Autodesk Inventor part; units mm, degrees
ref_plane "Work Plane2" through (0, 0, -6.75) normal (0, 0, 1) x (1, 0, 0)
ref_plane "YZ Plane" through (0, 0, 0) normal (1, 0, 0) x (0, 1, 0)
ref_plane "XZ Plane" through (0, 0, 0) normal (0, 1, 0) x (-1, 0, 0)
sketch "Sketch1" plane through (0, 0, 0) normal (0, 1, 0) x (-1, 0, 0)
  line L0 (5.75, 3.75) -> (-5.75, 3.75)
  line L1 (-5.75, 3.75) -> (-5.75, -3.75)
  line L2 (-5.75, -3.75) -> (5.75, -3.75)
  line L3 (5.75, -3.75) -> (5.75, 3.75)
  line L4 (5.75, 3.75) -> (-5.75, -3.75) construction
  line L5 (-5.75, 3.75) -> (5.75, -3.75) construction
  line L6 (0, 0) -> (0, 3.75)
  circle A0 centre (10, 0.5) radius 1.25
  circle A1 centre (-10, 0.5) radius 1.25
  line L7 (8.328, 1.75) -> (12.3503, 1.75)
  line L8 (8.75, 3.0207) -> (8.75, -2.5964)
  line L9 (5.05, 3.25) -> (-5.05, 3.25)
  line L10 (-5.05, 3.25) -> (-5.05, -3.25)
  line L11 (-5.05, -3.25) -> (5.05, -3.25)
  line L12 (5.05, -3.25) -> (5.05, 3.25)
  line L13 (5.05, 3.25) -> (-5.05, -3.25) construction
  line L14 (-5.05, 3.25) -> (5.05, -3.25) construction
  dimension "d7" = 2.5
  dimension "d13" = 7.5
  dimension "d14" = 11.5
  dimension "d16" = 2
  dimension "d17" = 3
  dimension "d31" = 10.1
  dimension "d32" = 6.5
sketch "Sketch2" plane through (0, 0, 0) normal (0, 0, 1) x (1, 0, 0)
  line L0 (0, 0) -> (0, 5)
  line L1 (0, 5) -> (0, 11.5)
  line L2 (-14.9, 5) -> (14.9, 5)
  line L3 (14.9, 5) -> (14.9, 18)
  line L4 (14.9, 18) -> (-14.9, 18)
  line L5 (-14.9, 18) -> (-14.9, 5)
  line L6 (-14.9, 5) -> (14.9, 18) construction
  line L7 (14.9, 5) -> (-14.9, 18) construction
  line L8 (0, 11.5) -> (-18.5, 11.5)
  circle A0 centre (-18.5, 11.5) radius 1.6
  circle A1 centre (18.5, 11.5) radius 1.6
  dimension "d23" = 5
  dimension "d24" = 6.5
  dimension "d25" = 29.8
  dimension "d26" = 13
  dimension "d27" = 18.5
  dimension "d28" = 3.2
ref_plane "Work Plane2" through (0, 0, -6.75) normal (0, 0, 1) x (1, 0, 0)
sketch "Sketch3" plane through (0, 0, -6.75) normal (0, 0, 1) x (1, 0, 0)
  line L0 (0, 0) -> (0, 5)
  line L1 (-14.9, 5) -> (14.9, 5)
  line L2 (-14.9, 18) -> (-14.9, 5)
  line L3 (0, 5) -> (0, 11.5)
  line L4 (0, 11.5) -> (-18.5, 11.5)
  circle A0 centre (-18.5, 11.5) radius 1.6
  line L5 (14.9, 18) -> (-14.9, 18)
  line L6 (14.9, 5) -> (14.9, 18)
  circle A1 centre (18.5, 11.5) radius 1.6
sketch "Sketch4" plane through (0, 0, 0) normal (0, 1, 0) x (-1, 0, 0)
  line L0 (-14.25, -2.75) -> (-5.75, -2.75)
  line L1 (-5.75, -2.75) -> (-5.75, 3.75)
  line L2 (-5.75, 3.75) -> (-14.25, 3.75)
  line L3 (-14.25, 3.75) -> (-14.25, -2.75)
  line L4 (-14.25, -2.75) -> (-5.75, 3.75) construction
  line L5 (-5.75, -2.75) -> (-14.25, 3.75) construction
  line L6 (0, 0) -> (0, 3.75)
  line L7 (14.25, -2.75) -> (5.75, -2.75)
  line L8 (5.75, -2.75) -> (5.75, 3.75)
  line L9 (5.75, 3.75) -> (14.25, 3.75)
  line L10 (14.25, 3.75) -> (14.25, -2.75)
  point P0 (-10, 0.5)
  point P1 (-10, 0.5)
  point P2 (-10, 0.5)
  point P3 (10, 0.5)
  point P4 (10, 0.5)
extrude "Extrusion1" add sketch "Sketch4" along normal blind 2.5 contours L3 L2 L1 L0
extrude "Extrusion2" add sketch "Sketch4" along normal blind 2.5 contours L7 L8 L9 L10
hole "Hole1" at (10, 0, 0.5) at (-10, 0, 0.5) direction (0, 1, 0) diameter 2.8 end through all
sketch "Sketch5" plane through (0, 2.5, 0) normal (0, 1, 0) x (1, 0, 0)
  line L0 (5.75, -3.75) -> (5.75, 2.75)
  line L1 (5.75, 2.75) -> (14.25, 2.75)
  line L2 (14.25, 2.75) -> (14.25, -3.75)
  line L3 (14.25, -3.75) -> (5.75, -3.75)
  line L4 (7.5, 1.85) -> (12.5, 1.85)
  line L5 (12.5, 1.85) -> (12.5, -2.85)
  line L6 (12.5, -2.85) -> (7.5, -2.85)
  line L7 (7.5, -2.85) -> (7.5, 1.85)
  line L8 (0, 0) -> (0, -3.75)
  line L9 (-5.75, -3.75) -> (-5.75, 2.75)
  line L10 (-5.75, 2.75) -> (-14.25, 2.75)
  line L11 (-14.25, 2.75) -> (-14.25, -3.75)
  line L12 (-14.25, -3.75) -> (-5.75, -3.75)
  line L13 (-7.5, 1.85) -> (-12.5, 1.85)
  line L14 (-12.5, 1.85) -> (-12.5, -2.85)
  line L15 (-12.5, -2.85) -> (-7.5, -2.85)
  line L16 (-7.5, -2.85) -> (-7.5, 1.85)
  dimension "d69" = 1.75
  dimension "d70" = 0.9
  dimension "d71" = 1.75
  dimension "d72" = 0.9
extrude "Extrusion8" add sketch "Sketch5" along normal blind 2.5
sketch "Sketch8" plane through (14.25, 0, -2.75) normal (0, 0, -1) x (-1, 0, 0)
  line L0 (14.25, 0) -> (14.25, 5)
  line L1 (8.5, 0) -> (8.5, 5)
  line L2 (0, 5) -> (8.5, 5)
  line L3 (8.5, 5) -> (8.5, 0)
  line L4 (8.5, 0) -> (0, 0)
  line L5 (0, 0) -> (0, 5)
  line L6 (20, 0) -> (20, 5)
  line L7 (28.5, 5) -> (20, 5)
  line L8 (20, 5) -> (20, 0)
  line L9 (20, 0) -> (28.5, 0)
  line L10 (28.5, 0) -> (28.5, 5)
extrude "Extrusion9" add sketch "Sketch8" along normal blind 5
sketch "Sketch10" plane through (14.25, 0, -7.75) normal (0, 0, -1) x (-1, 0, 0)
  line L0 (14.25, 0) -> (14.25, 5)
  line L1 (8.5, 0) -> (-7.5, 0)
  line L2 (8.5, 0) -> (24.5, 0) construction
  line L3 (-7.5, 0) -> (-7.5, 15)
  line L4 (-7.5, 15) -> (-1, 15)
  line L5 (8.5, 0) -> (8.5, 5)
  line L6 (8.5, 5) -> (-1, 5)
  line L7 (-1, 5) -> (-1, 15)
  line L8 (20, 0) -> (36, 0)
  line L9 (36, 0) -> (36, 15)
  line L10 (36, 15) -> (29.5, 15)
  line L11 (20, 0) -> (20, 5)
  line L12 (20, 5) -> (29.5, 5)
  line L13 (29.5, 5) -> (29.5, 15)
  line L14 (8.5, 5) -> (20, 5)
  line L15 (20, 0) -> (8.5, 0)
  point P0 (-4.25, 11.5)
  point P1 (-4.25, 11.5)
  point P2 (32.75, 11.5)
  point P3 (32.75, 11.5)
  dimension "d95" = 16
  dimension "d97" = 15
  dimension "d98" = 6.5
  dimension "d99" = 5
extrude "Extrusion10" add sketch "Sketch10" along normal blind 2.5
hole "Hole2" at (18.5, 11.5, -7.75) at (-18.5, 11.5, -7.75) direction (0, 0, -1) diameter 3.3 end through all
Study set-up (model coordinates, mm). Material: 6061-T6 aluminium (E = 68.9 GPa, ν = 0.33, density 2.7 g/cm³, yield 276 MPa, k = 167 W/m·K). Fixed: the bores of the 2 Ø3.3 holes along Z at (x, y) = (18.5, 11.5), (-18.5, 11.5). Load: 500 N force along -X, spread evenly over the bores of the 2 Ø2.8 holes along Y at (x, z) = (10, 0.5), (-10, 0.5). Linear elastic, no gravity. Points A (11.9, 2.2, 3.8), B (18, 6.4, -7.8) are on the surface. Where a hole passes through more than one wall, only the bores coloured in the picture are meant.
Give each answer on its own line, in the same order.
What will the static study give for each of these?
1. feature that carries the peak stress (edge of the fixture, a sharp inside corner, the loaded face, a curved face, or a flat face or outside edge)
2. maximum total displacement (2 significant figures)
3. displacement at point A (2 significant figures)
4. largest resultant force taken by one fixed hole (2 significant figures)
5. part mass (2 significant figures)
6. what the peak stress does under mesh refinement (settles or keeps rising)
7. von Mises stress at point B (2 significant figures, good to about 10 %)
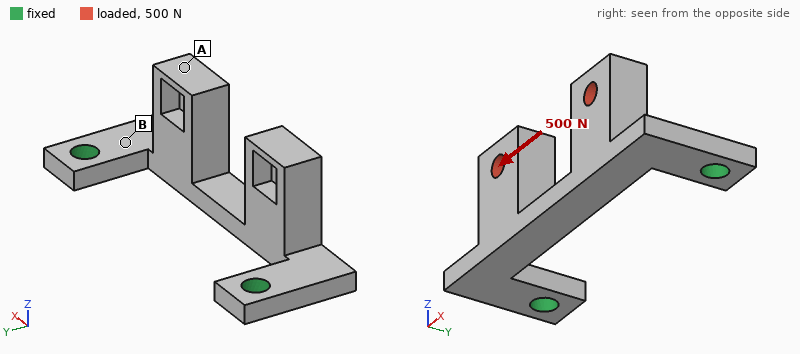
edge of the fixture
96 µm
90 µm
290 N
4.5 g
keeps rising
62 MPa
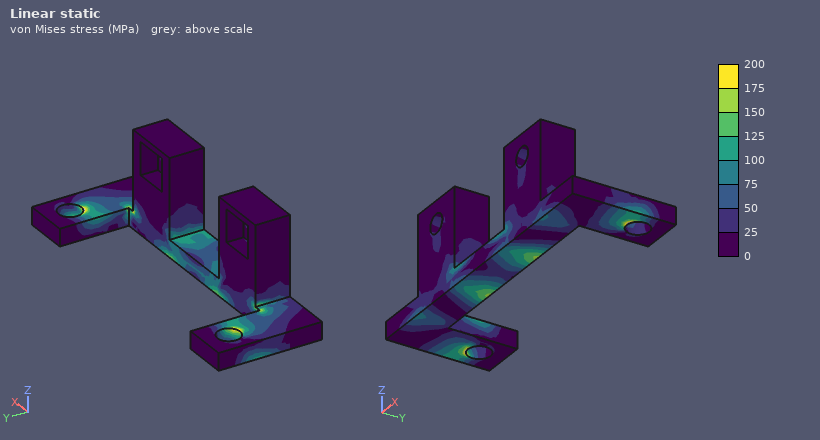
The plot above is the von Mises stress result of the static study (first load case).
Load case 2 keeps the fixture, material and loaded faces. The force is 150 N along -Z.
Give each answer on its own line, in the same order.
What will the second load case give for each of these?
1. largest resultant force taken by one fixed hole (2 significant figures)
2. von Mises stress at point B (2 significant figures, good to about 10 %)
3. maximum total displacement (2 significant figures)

75 N
75 MPa
0.14 mm
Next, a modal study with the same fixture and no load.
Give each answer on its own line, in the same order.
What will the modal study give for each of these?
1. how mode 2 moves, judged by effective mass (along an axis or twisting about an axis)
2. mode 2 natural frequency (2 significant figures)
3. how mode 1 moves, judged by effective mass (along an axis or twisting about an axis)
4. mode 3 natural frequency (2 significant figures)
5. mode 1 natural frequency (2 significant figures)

along Y
5000 Hz
along Z
6200 Hz
3400 Hz
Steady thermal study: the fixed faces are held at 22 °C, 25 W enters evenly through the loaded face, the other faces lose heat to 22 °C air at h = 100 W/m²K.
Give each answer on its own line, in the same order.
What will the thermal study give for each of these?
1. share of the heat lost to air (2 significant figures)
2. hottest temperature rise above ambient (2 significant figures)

26 %
65 K
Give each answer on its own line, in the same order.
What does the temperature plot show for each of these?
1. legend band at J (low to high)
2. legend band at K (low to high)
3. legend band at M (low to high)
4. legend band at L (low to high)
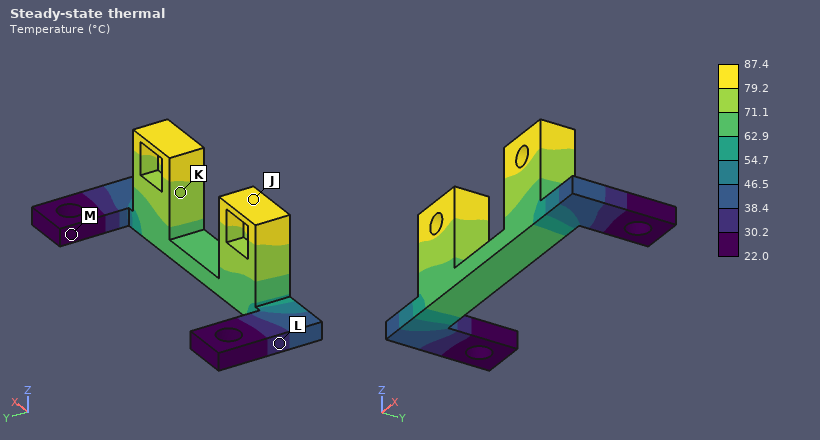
79.2 to 87.4 °C
71.1 to 79.2 °C
22.0 to 30.2 °C
30.2 to 38.4 °C
